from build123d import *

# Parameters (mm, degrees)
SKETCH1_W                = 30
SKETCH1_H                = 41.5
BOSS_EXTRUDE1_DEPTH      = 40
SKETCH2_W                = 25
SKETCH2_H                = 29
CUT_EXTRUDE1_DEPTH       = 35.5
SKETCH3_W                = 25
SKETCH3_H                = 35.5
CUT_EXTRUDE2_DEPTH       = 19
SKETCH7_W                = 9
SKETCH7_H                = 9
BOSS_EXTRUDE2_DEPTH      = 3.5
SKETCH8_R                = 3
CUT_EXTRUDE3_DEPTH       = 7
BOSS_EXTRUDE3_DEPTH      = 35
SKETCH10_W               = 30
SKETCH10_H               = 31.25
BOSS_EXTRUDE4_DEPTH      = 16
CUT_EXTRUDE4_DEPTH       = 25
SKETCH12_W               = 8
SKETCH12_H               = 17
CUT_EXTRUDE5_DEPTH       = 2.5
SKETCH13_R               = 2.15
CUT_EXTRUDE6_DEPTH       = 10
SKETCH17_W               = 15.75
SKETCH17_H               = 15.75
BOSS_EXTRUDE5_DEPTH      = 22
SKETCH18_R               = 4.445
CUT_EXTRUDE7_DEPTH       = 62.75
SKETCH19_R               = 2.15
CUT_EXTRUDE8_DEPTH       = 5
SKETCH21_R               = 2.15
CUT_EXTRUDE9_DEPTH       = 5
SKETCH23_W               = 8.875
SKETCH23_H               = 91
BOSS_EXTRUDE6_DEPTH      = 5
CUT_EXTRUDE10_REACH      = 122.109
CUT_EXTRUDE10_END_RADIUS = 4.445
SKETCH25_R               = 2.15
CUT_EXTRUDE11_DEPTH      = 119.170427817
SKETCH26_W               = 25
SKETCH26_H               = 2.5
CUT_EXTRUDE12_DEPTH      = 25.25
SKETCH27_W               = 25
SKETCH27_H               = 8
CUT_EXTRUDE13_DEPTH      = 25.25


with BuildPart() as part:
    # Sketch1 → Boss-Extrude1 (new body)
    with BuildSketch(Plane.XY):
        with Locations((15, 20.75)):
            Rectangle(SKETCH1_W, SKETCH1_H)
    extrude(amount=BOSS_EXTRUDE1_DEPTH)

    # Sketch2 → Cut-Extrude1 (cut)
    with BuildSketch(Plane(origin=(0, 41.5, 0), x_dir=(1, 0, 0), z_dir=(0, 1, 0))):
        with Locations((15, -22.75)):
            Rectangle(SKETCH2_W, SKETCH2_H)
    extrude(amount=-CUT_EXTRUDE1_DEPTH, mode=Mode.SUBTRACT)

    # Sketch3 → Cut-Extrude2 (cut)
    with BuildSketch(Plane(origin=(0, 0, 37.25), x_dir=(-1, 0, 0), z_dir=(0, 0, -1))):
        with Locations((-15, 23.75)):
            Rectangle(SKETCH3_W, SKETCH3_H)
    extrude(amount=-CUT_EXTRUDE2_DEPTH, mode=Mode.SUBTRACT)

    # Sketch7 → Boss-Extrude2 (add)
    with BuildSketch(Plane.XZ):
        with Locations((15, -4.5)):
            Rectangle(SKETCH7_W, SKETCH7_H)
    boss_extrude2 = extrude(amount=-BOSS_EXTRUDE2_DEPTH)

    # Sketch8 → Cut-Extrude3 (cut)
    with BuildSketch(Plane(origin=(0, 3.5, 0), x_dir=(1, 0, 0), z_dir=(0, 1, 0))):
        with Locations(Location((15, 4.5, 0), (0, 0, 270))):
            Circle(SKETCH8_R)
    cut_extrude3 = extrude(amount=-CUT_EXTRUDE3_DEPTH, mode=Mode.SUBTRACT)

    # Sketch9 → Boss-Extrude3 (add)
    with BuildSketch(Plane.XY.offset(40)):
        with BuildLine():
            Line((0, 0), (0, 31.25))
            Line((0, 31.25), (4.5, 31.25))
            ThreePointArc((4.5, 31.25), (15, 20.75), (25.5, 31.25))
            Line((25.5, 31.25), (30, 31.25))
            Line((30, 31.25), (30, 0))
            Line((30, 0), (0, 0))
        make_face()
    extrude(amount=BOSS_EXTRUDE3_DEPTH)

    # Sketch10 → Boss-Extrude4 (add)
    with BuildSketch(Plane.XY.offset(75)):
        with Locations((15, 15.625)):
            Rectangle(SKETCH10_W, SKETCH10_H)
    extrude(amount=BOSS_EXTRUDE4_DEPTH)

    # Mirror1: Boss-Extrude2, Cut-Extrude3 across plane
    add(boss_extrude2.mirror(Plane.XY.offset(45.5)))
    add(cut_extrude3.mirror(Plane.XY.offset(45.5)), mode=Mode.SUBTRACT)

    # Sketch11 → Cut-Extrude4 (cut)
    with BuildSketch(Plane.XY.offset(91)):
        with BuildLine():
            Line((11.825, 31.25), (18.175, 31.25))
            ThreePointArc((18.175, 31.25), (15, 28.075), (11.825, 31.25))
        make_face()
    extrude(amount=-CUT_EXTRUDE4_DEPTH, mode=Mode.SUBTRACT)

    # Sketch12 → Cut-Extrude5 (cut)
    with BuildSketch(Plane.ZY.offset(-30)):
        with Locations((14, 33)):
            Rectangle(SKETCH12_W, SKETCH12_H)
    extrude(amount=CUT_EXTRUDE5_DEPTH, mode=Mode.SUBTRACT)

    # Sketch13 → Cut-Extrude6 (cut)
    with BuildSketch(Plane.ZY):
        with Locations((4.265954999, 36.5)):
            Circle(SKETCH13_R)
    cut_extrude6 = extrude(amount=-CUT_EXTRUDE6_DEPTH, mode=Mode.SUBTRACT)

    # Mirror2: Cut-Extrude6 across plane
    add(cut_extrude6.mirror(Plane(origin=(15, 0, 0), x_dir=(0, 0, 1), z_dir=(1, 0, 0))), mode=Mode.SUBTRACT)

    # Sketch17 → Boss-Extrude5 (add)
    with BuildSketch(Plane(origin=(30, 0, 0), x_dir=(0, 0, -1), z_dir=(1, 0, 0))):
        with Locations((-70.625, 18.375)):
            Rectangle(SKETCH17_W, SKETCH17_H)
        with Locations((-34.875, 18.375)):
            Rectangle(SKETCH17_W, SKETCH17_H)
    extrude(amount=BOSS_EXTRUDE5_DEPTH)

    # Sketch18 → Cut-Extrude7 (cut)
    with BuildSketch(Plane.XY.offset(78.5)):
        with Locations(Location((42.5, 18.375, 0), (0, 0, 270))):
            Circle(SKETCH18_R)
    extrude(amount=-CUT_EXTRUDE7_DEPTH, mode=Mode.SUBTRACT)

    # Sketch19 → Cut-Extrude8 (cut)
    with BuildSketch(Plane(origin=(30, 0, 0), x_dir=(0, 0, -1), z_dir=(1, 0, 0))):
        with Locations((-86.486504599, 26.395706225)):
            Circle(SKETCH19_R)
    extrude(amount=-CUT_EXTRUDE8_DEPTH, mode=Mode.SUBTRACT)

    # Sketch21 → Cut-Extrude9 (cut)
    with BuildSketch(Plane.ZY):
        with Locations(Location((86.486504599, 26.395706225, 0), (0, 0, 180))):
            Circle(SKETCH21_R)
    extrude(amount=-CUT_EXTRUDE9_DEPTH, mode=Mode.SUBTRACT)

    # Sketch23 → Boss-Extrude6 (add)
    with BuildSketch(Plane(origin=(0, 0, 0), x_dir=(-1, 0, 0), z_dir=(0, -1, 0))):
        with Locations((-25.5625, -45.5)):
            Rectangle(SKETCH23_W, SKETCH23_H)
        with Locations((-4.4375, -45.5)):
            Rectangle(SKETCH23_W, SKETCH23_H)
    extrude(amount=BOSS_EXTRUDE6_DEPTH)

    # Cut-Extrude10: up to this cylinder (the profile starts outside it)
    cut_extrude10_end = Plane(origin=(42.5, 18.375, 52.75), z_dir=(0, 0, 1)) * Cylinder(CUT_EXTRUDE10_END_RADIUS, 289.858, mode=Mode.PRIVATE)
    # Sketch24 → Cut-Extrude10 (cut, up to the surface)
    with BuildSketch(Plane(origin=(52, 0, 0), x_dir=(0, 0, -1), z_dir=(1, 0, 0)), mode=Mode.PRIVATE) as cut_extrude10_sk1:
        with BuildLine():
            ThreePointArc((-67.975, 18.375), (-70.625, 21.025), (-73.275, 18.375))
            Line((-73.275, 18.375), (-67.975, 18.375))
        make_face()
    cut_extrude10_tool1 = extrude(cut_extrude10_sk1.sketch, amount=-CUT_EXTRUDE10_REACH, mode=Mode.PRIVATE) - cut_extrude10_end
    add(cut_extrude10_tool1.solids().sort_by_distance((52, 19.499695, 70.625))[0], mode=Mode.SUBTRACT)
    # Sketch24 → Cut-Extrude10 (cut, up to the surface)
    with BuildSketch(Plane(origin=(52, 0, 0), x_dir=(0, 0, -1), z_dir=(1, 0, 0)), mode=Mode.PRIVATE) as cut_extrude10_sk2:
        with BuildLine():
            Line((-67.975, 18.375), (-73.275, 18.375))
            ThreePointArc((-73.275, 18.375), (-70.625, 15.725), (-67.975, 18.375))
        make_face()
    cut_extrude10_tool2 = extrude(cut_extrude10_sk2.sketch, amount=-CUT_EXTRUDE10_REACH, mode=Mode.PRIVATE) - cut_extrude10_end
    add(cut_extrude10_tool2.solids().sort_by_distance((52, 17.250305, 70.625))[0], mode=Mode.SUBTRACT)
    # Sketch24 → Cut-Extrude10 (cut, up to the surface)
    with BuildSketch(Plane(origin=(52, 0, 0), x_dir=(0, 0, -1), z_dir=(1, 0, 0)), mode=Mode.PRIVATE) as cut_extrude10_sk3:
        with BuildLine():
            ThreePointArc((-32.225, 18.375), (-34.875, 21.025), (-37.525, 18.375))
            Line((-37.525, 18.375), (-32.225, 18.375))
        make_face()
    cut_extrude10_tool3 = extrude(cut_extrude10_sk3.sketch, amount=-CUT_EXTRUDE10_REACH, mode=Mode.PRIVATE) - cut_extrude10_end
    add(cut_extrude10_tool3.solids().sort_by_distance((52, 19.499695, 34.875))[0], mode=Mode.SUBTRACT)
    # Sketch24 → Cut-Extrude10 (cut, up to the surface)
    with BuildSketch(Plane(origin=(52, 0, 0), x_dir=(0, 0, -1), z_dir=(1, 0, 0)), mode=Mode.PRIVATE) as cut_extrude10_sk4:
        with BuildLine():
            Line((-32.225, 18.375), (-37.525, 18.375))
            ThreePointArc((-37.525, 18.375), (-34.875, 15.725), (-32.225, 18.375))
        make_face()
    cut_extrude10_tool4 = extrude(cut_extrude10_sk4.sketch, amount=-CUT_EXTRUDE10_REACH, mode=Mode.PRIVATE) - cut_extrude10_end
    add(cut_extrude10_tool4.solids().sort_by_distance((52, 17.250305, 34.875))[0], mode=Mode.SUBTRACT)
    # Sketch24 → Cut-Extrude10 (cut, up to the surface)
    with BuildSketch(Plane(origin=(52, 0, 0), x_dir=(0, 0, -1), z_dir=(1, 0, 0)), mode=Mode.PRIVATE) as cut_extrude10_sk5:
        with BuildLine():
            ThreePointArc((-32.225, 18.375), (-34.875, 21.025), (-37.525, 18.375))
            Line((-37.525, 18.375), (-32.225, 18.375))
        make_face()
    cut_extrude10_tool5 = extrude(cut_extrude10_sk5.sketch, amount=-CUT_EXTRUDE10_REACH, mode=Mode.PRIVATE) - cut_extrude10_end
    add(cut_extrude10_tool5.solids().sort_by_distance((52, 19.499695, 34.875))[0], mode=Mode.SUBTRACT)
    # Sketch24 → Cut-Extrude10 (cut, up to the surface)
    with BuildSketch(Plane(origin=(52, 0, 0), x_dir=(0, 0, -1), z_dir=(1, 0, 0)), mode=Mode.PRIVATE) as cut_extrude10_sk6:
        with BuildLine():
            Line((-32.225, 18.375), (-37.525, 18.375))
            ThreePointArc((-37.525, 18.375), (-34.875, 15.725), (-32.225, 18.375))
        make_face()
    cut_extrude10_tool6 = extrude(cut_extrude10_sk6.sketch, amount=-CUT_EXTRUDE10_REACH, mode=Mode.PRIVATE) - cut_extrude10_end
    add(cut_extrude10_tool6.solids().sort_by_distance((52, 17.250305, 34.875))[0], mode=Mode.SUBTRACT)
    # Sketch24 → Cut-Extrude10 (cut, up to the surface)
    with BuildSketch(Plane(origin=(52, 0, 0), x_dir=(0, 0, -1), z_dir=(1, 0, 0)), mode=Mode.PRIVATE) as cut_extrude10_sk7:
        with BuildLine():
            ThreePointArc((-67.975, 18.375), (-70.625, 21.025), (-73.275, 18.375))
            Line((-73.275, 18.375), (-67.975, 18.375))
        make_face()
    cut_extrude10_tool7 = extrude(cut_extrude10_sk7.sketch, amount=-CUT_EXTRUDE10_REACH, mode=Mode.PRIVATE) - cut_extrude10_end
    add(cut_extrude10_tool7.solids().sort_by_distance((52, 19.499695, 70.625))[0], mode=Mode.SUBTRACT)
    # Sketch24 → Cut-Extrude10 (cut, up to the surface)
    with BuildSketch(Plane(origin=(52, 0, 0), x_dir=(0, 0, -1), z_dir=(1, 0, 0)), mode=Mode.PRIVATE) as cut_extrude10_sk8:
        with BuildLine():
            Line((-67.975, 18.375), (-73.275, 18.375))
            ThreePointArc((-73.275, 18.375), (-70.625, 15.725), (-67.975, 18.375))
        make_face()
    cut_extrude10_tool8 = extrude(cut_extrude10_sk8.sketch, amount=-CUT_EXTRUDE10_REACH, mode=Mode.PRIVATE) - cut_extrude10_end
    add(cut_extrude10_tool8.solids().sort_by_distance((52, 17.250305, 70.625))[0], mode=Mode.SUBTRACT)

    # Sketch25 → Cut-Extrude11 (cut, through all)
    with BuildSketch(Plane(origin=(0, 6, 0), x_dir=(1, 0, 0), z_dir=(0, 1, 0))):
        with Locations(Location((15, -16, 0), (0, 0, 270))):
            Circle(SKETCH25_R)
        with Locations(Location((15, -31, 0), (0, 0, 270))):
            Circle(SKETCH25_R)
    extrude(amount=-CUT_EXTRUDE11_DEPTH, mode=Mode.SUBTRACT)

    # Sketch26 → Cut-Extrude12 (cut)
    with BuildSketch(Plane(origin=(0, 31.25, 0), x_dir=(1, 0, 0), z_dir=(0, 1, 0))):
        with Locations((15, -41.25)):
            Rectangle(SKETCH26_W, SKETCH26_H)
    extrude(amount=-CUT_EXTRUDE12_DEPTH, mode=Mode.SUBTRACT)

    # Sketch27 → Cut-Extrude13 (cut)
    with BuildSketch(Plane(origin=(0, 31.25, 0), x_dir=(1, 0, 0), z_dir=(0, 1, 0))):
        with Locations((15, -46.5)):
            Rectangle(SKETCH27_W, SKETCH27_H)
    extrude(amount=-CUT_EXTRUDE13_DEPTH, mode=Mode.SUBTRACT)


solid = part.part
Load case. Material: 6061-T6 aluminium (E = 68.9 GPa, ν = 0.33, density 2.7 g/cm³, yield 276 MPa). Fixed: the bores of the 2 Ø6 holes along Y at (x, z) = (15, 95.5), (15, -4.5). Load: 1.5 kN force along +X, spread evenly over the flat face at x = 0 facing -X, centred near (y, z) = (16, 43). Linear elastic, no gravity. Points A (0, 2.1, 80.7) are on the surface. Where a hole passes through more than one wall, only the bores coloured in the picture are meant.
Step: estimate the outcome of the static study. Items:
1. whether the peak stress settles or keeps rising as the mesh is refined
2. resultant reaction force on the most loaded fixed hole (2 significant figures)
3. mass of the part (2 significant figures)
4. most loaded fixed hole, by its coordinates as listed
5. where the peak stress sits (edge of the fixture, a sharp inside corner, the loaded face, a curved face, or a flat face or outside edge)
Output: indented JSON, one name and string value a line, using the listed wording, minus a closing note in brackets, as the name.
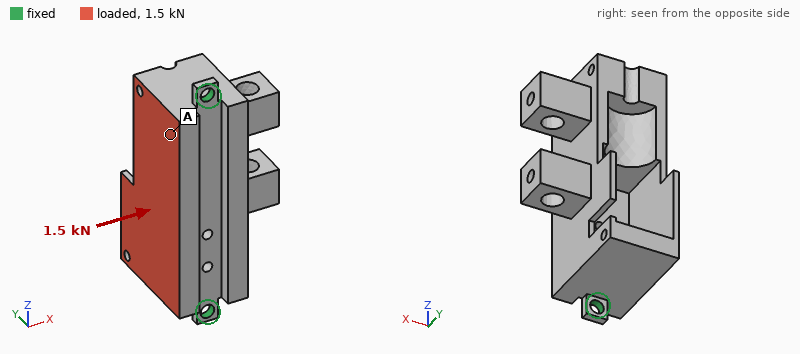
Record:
{
  "whether the peak stress settles or keeps rising as the mesh is refined": "keeps rising",
  "resultant reaction force on the most loaded fixed hole": "790 N",
  "mass of the part": "200 g",
  "most loaded fixed hole, by its coordinates as listed": "(15, -4.5)",
  "where the peak stress sits": "edge of the fixture"
}
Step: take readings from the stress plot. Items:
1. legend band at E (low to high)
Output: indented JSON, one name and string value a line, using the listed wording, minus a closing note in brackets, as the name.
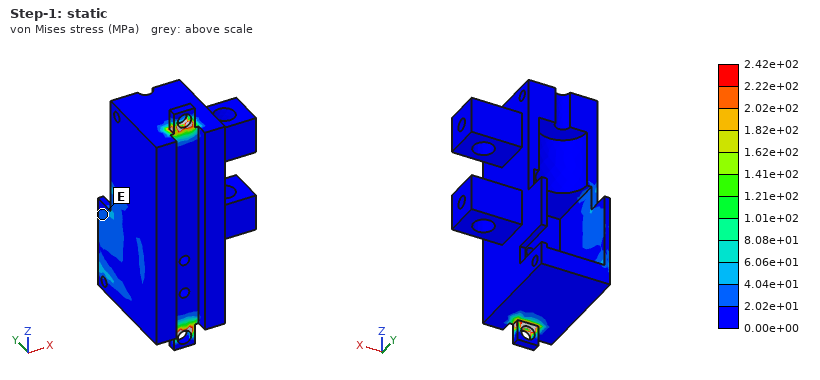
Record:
{
  "legend band at E": "2.02e+01 to 4.04e+01 MPa"
}
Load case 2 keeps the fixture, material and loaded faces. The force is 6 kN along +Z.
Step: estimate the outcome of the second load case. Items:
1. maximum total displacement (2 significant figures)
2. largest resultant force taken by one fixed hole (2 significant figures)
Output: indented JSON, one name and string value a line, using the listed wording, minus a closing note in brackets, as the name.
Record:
{
  "maximum total displacement": "41 µm",
  "largest resultant force taken by one fixed hole": "3.5 kN"
}
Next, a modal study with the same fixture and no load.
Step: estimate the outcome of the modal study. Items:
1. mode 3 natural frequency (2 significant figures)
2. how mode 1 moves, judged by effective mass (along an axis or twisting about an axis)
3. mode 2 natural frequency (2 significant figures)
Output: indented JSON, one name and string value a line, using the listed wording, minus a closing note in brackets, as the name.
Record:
{
  "mode 3 natural frequency": "3600 Hz",
  "how mode 1 moves, judged by effective mass": "along X",
  "mode 2 natural frequency": "3400 Hz"
}
